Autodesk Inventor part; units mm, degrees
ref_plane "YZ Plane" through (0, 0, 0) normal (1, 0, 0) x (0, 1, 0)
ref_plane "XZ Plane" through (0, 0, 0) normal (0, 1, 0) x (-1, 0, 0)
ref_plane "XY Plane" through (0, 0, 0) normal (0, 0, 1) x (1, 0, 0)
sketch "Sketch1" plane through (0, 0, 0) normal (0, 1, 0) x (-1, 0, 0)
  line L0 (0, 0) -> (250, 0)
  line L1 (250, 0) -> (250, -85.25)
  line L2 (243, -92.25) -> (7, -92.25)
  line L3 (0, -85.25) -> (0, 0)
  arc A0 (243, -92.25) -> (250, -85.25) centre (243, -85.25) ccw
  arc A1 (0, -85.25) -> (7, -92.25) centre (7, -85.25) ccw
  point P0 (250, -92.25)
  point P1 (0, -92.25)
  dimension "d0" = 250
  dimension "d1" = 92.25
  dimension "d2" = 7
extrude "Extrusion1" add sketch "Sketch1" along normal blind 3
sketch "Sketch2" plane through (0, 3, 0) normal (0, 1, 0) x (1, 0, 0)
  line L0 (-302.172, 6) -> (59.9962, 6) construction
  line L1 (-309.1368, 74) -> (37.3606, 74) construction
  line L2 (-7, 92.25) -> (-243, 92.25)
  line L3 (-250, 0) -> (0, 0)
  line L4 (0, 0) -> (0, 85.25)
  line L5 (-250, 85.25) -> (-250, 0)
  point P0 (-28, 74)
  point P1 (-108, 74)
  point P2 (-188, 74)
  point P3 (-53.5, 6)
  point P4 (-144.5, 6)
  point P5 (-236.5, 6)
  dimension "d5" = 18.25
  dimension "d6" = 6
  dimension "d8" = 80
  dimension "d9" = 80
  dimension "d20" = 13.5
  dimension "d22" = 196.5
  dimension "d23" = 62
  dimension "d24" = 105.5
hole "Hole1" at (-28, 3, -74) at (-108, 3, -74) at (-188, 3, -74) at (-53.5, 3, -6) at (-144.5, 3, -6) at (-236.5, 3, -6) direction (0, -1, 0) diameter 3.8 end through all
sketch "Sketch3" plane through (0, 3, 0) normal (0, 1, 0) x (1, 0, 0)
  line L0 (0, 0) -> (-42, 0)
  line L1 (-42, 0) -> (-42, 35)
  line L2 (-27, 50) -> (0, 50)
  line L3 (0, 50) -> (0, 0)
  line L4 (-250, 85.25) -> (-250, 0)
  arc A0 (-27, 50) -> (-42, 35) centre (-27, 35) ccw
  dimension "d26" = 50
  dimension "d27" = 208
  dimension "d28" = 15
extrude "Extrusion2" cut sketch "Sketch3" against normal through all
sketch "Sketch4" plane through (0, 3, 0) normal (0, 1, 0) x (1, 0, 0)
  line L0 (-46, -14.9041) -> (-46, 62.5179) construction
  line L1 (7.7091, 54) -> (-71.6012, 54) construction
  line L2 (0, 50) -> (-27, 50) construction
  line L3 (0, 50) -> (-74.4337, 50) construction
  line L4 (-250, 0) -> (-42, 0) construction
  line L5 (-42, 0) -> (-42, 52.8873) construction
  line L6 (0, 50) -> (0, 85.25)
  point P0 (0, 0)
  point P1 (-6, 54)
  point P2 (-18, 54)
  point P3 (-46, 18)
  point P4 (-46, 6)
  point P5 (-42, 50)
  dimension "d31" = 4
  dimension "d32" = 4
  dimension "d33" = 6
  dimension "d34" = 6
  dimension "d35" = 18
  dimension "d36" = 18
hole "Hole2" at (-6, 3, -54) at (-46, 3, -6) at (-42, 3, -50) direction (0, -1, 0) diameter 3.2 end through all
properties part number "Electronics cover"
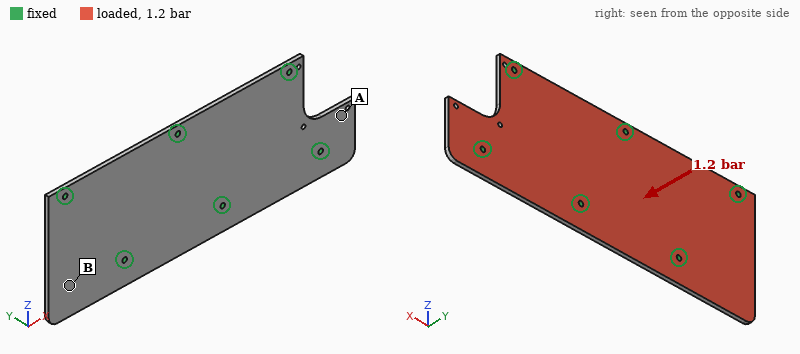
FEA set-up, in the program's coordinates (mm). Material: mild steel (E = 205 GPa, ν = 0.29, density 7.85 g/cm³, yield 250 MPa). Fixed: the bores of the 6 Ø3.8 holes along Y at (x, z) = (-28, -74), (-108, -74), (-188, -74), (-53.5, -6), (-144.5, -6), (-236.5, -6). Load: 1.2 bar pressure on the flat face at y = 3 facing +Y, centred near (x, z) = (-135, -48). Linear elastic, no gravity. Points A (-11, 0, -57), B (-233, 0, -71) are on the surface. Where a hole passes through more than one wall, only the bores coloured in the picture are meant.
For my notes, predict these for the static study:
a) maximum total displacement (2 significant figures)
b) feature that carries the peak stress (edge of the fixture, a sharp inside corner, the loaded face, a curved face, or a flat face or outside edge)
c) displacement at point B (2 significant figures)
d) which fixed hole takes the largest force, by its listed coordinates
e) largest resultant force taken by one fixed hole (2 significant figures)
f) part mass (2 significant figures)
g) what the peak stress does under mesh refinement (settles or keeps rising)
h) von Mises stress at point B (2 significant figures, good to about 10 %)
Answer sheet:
0.26 mm
edge of the fixture
0.16 mm
(-188, -74)
620 N
490 g
keeps rising
28 MPa
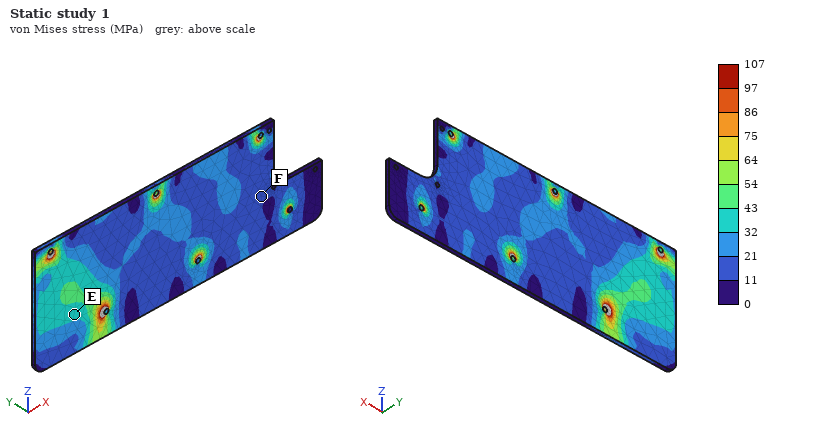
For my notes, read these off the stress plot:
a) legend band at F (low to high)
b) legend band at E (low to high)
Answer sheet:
11 to 21 MPa
32 to 43 MPa
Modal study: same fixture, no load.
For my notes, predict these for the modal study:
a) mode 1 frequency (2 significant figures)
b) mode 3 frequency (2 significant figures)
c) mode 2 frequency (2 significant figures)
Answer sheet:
920 Hz
1800 Hz
1800 Hz
